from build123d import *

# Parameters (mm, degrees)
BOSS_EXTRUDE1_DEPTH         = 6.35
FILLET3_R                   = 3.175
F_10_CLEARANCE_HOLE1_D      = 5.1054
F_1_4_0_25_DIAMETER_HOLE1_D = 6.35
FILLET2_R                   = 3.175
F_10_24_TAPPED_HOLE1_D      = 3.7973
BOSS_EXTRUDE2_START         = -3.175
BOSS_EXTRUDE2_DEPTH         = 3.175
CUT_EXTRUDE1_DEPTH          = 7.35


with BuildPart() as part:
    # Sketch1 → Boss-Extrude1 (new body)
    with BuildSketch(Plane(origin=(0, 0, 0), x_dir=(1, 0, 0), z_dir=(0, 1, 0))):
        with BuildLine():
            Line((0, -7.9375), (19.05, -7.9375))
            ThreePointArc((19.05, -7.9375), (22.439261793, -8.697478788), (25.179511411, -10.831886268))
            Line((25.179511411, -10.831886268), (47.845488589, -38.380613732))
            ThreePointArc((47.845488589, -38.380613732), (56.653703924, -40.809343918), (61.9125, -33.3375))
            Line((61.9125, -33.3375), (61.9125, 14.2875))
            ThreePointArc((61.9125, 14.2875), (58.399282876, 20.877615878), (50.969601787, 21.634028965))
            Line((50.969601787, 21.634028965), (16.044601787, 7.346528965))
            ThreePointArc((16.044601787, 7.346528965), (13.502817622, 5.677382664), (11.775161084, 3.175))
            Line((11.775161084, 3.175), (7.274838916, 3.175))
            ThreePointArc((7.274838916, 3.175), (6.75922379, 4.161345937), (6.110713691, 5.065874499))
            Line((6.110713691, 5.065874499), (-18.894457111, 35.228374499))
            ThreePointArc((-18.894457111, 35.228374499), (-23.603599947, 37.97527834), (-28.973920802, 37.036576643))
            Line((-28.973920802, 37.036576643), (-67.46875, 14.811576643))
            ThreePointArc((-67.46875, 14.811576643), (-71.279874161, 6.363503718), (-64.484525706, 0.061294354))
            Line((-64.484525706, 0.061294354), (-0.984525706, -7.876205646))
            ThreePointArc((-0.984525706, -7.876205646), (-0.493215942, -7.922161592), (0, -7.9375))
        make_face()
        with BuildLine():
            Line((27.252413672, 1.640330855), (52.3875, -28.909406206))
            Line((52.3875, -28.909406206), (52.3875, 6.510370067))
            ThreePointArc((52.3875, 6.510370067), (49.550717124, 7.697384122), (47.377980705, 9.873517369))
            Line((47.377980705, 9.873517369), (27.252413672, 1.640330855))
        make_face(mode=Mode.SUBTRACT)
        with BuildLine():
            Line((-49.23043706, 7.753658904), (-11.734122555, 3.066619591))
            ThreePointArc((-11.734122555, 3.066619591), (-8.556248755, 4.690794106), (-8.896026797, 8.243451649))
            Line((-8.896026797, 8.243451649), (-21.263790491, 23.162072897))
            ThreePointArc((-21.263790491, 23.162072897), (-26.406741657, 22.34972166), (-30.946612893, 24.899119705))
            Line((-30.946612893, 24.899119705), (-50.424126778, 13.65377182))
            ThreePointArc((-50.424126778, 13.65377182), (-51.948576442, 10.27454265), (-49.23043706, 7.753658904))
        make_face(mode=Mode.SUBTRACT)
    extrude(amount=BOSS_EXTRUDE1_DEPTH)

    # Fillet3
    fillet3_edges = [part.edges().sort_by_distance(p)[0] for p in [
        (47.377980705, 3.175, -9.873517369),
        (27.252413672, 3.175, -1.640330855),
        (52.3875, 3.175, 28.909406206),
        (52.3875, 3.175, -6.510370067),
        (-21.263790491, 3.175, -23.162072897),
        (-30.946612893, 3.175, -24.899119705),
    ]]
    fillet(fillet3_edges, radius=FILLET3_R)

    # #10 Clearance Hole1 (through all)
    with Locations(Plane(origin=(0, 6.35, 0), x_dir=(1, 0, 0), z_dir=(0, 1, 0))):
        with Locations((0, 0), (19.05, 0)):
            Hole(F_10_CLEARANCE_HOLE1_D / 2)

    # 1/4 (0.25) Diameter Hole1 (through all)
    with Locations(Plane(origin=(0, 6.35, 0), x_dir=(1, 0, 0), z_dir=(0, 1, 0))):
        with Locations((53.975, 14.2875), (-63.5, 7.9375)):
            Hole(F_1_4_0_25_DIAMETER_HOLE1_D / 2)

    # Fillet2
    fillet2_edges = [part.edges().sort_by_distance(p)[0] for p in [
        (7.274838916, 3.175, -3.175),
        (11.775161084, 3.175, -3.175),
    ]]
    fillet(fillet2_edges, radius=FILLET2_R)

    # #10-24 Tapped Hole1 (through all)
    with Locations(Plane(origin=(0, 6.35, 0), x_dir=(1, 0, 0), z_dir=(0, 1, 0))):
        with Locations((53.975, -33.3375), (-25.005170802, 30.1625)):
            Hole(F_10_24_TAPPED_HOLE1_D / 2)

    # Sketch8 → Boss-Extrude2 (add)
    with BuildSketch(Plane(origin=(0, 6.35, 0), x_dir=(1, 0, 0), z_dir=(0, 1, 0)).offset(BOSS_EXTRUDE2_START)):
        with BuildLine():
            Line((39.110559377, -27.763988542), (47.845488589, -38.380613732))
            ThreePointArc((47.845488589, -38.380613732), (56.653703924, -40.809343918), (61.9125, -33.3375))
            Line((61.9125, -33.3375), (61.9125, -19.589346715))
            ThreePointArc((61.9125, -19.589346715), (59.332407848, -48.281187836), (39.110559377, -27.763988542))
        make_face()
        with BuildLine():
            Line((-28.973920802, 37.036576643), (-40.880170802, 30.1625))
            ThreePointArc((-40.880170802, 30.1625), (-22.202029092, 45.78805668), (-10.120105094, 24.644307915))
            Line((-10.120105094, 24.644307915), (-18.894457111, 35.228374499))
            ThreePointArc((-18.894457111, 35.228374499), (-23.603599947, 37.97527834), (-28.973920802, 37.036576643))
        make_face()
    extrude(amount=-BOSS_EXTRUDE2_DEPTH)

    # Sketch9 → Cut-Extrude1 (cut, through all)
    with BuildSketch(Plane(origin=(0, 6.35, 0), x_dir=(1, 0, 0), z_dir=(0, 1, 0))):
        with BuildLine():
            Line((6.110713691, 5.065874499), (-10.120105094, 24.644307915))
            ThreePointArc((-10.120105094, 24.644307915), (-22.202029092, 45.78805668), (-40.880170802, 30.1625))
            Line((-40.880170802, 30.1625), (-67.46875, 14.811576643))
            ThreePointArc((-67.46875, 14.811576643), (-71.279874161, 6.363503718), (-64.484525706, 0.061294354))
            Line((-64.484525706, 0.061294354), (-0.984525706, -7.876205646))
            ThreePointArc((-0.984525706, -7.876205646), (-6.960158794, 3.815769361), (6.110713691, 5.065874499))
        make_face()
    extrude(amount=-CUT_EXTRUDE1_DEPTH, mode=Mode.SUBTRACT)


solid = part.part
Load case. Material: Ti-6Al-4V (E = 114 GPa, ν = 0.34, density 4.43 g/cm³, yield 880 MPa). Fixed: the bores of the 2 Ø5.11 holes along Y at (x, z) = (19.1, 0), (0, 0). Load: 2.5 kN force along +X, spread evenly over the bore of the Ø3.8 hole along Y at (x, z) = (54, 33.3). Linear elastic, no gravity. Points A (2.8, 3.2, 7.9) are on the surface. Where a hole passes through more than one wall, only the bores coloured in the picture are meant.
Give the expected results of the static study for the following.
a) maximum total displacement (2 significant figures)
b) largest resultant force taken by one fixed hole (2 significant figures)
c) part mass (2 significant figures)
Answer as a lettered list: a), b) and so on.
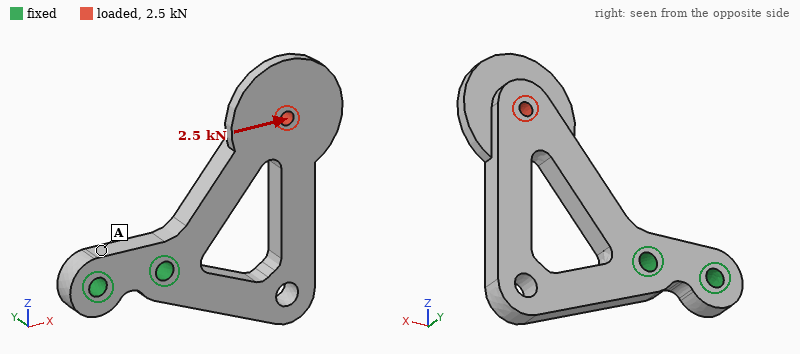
a) 0.56 mm
b) 2.4 kN
c) 53 g
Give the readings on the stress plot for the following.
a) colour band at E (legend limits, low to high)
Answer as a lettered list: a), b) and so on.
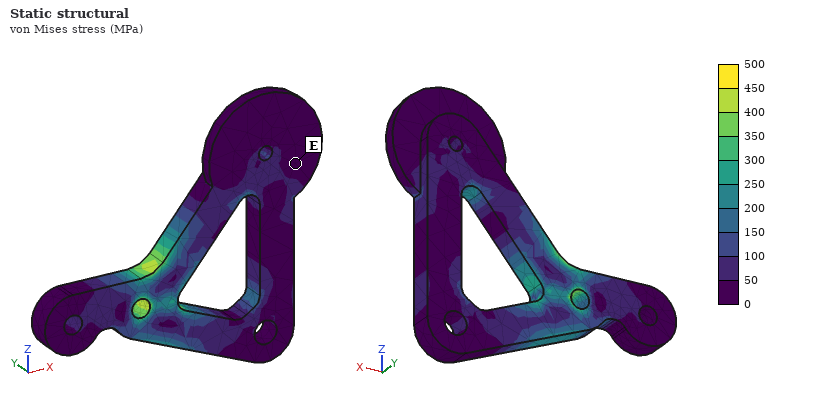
a) 0 to 50 MPa
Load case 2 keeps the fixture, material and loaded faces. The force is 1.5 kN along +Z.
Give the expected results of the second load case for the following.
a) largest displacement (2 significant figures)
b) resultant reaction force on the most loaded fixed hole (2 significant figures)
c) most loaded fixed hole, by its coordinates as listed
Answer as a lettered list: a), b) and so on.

a) 0.33 mm
b) 2.8 kN
c) (19.1, 0)
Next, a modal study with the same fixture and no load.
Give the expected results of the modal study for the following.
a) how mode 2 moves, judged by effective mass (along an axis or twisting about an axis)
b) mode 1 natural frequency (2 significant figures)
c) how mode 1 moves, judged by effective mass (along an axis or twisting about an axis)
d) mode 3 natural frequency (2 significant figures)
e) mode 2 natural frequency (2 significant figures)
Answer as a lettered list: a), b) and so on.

a) along Z
b) 1200 Hz
c) along Y
d) 2300 Hz
e) 2100 Hz
